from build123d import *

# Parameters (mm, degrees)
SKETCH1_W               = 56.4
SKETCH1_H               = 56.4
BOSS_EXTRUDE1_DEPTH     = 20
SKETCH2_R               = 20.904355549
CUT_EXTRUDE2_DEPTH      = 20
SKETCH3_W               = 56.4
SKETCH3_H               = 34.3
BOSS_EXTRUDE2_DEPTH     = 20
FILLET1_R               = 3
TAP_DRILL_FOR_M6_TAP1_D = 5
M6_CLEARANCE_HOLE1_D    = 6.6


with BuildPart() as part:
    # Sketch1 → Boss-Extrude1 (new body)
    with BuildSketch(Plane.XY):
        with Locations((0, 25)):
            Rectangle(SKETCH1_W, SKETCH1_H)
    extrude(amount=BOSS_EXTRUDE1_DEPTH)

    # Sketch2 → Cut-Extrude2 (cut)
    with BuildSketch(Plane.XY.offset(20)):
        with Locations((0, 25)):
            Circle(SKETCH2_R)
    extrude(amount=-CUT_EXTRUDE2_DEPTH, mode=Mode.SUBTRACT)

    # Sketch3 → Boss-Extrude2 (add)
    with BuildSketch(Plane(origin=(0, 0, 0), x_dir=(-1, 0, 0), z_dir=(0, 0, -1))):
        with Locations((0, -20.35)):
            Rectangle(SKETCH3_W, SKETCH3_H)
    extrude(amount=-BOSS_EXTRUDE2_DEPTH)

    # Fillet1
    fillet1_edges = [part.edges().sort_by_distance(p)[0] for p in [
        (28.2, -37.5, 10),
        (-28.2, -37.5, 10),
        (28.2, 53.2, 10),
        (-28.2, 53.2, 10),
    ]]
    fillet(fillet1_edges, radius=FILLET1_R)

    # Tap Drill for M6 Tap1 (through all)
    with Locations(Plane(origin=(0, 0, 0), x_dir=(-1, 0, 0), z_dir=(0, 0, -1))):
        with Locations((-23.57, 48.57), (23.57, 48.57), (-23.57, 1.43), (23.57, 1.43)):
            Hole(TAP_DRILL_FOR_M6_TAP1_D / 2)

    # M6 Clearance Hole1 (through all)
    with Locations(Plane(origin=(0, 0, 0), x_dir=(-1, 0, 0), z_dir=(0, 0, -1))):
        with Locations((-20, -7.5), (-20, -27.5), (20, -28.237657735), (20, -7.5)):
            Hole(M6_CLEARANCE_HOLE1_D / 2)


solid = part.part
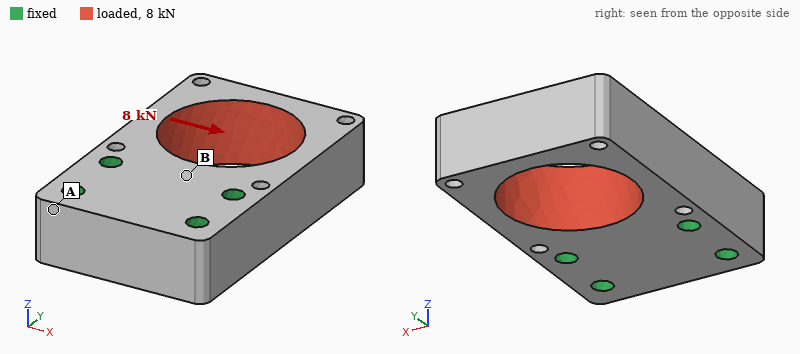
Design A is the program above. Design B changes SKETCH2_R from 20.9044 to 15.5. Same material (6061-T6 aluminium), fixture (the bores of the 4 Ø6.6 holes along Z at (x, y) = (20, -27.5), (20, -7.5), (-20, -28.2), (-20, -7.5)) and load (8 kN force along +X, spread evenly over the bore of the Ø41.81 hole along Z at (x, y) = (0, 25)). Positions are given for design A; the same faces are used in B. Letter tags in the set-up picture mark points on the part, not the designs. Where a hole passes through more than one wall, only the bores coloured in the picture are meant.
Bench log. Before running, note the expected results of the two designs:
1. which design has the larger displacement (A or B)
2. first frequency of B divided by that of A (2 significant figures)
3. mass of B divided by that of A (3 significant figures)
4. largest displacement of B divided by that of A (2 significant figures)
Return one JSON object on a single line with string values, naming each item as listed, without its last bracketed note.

{"which design has the larger displacement": "A", "first frequency of B divided by that of A": "1.1", "mass of B divided by that of A": "1.18", "largest displacement of B divided by that of A": "0.37"}
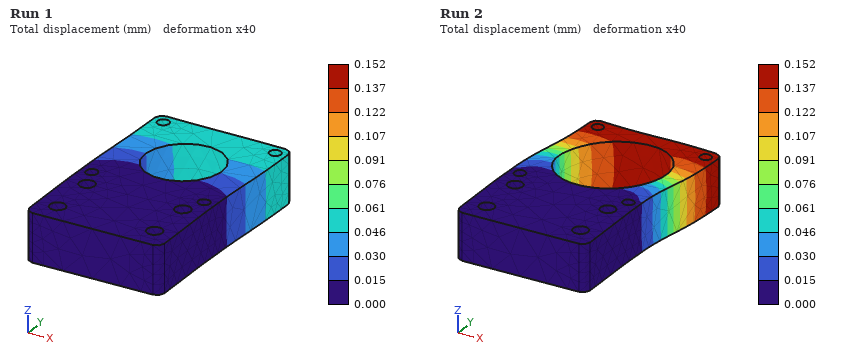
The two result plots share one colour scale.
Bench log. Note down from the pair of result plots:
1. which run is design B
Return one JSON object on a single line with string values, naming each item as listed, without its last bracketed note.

{"which run is design B": "Run 1"}
